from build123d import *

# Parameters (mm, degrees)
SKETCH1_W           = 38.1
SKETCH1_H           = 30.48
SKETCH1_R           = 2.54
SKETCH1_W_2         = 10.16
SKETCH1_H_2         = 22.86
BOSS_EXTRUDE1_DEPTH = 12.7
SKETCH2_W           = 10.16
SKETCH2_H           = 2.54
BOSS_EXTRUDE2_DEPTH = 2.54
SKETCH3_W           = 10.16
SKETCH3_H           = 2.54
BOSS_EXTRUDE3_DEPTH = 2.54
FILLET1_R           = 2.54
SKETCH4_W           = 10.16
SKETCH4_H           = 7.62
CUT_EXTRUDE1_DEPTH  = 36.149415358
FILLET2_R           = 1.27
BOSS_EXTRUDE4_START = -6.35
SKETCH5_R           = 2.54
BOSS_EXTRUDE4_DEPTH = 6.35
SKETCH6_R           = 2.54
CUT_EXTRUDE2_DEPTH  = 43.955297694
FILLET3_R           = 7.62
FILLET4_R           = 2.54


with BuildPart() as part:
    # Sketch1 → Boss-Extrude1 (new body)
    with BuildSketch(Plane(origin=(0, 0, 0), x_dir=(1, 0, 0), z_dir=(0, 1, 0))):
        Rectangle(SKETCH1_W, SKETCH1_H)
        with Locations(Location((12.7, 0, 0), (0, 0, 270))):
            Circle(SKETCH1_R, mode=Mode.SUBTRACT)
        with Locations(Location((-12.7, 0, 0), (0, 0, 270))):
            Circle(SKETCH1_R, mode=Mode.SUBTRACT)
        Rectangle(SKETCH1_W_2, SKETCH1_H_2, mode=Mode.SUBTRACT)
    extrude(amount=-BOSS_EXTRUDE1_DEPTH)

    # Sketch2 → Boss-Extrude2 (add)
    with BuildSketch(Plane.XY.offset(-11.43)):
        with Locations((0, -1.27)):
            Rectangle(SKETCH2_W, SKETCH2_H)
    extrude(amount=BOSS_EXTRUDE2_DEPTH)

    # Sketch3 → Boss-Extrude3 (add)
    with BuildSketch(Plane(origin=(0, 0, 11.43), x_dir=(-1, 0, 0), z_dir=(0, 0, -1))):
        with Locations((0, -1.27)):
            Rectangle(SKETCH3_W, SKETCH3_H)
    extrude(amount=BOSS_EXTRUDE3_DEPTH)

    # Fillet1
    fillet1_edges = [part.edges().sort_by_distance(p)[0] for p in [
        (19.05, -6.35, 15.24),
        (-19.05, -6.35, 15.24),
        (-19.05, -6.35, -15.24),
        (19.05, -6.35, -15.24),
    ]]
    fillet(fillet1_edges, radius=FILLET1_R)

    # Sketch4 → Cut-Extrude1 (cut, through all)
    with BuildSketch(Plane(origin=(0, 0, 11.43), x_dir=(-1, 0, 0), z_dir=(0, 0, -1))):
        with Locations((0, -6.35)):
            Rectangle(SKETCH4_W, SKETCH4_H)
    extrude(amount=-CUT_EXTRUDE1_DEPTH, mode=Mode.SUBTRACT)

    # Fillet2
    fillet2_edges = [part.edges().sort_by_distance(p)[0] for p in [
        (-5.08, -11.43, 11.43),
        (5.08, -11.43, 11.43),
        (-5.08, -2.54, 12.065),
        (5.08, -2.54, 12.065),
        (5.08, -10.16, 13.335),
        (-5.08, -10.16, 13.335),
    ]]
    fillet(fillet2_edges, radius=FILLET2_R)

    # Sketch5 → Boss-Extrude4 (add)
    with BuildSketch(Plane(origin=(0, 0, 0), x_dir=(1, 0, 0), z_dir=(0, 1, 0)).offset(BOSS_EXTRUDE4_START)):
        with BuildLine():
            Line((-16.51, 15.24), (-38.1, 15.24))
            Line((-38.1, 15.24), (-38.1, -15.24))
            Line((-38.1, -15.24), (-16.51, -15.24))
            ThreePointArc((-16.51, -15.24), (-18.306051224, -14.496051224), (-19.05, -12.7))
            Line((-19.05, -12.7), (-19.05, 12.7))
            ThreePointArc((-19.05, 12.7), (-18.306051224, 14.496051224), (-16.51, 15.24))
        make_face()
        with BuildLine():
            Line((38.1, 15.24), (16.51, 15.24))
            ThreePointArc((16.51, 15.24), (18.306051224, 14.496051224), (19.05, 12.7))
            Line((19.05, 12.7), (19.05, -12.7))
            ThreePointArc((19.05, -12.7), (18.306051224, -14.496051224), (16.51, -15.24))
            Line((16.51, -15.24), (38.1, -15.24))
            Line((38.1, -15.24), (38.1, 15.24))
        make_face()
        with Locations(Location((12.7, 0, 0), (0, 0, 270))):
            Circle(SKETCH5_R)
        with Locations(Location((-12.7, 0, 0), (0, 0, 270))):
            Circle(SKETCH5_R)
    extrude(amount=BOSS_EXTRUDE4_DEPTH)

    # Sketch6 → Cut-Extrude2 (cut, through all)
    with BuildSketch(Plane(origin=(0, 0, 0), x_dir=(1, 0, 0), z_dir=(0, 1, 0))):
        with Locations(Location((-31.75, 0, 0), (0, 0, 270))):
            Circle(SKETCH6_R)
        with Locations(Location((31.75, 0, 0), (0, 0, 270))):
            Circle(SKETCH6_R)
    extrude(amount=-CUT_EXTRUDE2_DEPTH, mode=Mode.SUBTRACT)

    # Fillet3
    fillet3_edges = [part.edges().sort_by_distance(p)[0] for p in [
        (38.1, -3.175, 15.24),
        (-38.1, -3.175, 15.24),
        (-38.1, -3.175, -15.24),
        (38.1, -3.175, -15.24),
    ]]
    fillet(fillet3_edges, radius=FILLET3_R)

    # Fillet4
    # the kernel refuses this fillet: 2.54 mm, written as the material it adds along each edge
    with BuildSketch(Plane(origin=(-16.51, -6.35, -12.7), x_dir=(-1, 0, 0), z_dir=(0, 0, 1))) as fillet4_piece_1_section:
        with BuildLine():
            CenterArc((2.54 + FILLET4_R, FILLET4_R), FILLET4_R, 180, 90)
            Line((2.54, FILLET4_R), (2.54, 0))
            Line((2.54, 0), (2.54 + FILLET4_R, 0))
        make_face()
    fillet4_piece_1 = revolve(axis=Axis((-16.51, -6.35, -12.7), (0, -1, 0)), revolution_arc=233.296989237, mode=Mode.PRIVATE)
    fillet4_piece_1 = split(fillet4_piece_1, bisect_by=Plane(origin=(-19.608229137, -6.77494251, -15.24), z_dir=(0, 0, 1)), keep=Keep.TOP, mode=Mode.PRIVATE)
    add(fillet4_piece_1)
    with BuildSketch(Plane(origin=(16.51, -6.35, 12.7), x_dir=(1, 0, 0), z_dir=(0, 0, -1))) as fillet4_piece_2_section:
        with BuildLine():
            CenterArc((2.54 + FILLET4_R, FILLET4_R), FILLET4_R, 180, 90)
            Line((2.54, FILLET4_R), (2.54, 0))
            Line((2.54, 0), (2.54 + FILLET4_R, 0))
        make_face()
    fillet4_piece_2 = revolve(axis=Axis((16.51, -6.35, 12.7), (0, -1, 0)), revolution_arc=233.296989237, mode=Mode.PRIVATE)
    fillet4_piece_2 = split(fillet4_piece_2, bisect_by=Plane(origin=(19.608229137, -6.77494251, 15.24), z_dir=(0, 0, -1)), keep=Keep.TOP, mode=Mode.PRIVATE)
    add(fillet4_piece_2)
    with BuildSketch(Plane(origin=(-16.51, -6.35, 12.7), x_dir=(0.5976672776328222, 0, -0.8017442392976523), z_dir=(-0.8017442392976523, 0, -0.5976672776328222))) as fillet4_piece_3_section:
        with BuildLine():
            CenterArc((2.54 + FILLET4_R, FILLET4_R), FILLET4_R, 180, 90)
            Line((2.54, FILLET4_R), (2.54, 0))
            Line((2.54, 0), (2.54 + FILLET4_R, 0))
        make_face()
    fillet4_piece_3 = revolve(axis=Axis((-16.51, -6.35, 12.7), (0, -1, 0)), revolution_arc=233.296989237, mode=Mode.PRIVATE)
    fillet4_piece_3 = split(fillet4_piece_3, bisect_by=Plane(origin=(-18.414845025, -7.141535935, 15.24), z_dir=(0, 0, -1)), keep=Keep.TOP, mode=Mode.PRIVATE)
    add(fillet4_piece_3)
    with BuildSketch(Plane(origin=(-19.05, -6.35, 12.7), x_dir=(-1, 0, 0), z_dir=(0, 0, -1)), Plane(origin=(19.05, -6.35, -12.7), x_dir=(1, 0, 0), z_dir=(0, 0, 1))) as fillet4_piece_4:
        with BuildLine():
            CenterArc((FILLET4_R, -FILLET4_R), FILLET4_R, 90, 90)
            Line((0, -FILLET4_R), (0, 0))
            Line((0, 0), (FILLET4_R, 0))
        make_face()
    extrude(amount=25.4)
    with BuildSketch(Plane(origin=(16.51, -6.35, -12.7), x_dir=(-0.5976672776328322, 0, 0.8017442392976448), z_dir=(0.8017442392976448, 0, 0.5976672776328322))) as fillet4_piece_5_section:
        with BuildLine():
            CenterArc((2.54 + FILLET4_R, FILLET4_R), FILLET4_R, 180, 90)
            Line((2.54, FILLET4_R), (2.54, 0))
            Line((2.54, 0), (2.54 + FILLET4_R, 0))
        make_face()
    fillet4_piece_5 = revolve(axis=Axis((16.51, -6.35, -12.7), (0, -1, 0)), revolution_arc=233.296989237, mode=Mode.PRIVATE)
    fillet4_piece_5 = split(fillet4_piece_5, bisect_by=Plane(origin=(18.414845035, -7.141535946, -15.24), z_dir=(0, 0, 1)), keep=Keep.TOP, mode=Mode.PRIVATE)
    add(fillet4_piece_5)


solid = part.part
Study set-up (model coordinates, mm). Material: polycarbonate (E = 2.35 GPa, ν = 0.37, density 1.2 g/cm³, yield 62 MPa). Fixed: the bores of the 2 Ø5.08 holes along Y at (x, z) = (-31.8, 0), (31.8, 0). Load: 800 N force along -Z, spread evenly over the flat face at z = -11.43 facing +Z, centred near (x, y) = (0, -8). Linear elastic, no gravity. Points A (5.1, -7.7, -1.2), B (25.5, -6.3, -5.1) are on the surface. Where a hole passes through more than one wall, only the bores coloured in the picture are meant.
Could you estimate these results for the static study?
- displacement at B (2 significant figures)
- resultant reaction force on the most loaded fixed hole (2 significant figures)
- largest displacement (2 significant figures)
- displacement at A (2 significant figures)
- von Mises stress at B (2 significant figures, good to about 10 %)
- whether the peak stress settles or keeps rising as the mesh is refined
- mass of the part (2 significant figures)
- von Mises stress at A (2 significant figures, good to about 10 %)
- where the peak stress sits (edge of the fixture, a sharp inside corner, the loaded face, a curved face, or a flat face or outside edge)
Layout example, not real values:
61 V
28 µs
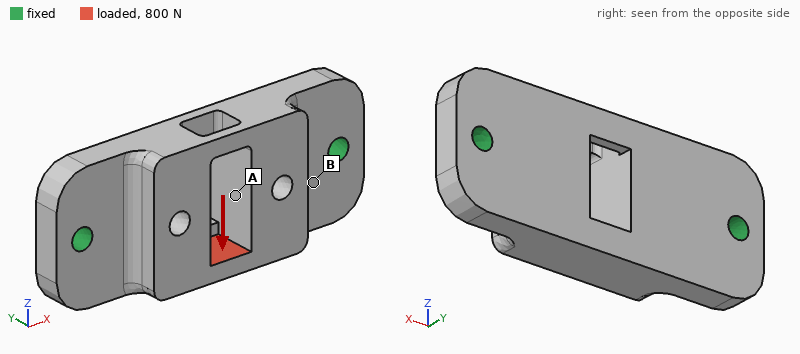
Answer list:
0.073 mm
420 N
0.48 mm
0.20 mm
11 MPa
keeps rising
22 g
4.3 MPa
edge of the fixture
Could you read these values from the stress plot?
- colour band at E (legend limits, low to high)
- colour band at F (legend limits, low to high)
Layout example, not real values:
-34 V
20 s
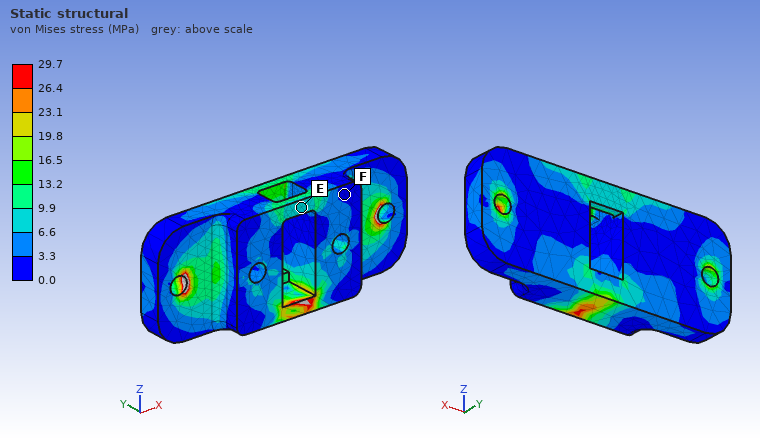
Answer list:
6.6 to 9.9 MPa
0.0 to 3.3 MPa
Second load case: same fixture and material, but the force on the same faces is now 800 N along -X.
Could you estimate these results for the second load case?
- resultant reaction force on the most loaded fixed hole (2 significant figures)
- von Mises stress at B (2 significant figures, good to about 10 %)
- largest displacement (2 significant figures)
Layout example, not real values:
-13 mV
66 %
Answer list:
420 N
5.6 MPa
0.16 mm
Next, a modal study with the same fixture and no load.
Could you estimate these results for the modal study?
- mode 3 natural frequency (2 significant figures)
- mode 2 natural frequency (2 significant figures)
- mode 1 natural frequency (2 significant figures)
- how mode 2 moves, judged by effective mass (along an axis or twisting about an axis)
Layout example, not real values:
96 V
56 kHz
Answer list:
3200 Hz
2100 Hz
2000 Hz
along Y
